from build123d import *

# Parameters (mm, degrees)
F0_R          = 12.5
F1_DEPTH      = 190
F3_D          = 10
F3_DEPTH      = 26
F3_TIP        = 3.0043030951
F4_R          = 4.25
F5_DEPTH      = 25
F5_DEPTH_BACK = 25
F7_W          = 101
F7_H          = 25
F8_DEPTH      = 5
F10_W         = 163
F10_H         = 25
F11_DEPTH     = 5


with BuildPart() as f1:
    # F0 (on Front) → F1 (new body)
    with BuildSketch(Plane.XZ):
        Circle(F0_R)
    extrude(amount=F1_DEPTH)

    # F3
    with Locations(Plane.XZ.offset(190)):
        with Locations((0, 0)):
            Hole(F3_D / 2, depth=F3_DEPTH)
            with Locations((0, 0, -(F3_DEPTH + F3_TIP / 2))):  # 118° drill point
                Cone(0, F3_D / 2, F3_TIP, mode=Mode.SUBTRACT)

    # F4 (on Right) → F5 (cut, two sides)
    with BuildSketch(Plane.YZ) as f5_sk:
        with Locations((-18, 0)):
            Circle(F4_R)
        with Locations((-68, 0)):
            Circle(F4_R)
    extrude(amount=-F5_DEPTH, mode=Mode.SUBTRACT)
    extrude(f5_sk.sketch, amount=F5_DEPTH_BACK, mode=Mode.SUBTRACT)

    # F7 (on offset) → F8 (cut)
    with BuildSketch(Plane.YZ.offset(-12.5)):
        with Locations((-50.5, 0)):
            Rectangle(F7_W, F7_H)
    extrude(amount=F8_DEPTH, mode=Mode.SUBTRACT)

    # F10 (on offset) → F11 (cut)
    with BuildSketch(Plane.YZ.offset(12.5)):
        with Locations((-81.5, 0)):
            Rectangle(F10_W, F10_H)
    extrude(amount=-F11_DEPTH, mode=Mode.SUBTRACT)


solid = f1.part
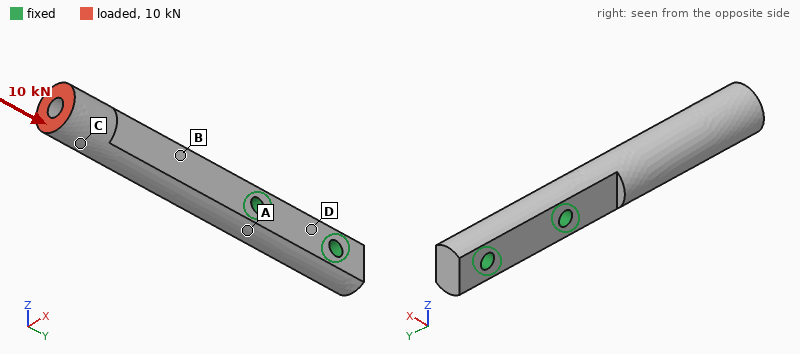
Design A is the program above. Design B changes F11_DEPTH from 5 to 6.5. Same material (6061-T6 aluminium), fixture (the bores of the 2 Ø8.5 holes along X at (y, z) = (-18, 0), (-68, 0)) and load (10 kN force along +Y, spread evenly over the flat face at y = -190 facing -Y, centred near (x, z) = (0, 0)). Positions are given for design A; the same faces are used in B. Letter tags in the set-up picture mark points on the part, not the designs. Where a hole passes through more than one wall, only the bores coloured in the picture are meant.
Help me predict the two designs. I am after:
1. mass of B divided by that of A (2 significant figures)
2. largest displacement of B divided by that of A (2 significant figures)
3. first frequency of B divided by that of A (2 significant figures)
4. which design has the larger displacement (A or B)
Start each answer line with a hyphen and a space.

- 0.93
- 2.4
- 0.88
- B
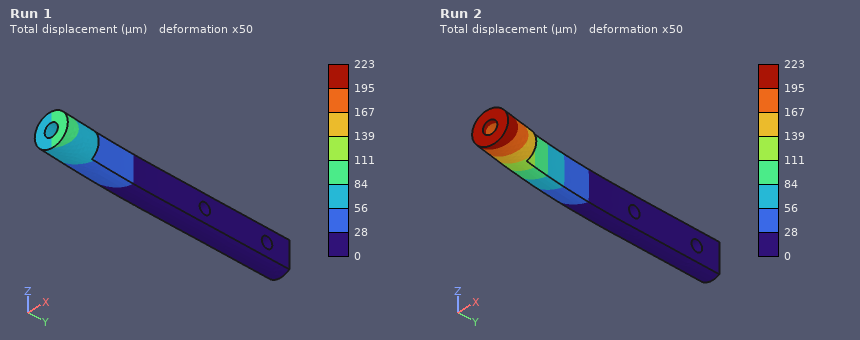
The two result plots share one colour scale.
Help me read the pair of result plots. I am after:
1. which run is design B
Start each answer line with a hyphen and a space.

- Run 2
